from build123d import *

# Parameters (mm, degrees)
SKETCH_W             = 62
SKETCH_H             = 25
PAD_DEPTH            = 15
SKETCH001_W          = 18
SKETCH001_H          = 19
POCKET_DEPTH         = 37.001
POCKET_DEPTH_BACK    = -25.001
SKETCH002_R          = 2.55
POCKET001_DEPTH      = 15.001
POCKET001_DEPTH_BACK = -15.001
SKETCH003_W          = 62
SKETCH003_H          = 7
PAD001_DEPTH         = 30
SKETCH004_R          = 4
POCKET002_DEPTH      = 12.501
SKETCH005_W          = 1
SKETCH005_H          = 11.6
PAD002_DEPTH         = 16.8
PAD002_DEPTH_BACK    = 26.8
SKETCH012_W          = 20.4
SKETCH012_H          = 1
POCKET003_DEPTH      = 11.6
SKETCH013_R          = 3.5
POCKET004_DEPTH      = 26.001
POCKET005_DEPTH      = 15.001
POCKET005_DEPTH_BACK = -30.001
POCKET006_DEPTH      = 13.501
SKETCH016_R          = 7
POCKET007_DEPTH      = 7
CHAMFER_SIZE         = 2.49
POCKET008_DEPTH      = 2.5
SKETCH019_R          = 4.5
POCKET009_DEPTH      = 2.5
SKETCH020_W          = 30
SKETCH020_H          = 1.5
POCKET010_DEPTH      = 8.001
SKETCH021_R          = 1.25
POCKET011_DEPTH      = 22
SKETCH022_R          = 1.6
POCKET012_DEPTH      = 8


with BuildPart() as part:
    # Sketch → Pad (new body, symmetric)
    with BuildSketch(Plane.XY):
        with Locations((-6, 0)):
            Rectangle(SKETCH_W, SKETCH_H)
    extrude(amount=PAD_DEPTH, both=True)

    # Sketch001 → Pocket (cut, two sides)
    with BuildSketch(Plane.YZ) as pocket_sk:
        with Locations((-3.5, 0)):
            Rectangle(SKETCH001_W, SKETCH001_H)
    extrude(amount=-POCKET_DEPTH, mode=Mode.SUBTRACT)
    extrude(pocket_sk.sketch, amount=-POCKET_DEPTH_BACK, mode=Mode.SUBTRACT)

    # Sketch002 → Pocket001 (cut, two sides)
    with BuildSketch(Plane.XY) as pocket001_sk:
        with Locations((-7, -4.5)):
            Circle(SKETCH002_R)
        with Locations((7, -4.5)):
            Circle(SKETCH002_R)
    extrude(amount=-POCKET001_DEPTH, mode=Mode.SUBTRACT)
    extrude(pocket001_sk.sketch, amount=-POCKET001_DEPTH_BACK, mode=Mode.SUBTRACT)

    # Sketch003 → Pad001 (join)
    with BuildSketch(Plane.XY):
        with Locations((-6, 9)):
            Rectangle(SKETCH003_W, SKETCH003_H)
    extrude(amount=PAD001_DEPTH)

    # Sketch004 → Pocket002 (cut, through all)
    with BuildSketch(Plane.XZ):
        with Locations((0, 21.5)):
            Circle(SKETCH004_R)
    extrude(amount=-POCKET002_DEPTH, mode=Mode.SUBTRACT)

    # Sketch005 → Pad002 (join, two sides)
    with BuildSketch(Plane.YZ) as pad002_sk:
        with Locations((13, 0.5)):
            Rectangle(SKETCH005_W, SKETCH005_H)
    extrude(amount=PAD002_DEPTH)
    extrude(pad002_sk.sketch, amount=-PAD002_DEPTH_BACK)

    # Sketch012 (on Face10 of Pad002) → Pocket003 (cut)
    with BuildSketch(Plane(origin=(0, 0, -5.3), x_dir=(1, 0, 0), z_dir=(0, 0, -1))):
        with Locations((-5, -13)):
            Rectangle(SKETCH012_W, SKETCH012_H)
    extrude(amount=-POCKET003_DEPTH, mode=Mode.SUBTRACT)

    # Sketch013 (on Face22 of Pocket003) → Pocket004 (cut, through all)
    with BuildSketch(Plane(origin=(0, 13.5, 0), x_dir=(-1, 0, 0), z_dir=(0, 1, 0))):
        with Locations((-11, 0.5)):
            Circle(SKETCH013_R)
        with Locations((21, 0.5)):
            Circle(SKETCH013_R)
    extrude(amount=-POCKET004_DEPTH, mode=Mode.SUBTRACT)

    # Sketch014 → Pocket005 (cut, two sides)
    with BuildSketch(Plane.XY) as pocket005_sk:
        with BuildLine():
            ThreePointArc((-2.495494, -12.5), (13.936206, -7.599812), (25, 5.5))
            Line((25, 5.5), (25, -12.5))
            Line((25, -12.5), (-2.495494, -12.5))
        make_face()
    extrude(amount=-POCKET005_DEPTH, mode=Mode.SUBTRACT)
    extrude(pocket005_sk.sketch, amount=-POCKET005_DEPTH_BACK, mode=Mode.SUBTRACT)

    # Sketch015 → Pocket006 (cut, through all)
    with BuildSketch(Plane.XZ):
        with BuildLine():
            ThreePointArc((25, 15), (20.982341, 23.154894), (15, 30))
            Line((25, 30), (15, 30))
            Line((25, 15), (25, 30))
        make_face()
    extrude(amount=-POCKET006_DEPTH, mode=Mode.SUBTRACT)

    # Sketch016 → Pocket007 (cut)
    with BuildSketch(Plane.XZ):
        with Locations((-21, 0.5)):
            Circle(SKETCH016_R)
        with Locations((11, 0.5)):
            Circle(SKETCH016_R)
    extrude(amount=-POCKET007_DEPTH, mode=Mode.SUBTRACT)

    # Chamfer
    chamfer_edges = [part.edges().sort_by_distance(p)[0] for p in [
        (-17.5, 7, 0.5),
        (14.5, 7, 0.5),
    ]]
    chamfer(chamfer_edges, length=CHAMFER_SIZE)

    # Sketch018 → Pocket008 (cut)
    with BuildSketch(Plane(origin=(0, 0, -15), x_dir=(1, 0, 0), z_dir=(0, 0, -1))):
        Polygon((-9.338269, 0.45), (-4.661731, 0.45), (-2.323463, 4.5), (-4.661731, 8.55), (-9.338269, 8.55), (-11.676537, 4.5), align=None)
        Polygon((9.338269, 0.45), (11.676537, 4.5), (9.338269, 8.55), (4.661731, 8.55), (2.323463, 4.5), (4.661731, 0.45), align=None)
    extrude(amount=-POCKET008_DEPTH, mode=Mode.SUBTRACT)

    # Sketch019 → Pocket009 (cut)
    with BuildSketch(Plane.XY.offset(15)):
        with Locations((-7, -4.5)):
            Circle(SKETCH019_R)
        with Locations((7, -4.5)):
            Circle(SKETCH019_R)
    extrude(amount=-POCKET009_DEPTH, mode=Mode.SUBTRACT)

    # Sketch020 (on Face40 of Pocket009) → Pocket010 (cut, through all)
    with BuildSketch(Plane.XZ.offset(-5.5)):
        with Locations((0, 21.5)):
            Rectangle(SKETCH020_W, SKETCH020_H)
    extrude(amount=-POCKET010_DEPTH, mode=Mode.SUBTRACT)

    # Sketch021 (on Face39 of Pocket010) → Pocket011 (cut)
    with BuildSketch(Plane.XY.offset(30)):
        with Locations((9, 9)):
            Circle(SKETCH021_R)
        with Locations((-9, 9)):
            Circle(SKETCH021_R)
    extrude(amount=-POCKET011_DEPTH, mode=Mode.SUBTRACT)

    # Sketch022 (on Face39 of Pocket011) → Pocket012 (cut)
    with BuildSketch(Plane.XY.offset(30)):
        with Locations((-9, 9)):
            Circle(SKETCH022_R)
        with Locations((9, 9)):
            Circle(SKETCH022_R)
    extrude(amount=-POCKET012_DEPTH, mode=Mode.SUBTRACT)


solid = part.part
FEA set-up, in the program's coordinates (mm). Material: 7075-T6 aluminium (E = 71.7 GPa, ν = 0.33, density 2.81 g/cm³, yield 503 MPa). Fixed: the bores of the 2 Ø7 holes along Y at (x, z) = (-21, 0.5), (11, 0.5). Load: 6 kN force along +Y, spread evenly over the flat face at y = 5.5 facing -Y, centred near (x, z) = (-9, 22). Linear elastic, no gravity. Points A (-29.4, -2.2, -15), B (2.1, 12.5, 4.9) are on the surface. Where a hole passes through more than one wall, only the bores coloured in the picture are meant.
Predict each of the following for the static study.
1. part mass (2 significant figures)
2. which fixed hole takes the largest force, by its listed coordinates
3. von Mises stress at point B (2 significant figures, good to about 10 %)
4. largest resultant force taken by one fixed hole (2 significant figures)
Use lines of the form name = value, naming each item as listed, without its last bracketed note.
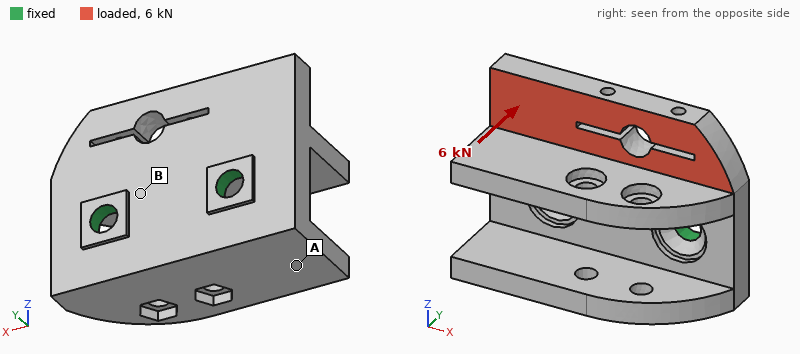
part mass = 77 g
which fixed hole takes the largest force, by its listed coordinates = (-21, 0.5)
von Mises stress at point B = 140 MPa
largest resultant force taken by one fixed hole = 3.6 kN
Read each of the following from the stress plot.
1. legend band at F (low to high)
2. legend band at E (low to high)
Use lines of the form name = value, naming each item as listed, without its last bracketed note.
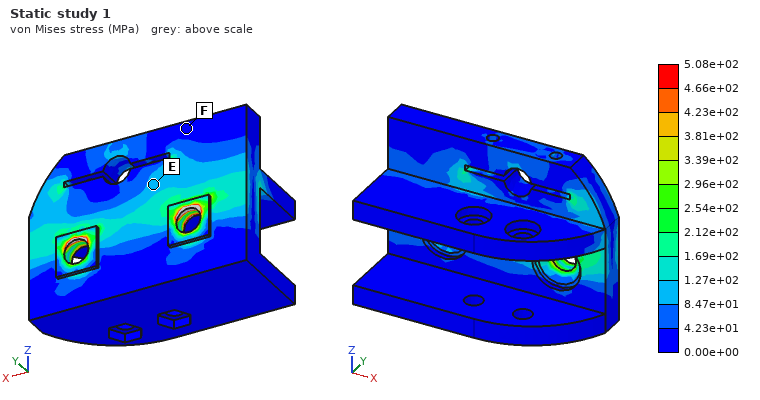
legend band at F = 0.00e+00 to 4.23e+01 MPa
legend band at E = 8.47e+01 to 1.27e+02 MPa
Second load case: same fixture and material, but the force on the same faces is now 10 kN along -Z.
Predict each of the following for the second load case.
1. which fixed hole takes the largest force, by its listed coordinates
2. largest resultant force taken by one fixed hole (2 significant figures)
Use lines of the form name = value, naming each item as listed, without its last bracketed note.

which fixed hole takes the largest force, by its listed coordinates = (-21, 0.5)
largest resultant force taken by one fixed hole = 6.1 kN
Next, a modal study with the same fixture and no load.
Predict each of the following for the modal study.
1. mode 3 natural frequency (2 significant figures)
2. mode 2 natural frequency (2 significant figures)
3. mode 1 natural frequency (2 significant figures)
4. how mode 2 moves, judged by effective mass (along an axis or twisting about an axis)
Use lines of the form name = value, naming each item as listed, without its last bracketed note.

mode 3 natural frequency = 7100 Hz
mode 2 natural frequency = 6500 Hz
mode 1 natural frequency = 3900 Hz
how mode 2 moves, judged by effective mass = along Y
